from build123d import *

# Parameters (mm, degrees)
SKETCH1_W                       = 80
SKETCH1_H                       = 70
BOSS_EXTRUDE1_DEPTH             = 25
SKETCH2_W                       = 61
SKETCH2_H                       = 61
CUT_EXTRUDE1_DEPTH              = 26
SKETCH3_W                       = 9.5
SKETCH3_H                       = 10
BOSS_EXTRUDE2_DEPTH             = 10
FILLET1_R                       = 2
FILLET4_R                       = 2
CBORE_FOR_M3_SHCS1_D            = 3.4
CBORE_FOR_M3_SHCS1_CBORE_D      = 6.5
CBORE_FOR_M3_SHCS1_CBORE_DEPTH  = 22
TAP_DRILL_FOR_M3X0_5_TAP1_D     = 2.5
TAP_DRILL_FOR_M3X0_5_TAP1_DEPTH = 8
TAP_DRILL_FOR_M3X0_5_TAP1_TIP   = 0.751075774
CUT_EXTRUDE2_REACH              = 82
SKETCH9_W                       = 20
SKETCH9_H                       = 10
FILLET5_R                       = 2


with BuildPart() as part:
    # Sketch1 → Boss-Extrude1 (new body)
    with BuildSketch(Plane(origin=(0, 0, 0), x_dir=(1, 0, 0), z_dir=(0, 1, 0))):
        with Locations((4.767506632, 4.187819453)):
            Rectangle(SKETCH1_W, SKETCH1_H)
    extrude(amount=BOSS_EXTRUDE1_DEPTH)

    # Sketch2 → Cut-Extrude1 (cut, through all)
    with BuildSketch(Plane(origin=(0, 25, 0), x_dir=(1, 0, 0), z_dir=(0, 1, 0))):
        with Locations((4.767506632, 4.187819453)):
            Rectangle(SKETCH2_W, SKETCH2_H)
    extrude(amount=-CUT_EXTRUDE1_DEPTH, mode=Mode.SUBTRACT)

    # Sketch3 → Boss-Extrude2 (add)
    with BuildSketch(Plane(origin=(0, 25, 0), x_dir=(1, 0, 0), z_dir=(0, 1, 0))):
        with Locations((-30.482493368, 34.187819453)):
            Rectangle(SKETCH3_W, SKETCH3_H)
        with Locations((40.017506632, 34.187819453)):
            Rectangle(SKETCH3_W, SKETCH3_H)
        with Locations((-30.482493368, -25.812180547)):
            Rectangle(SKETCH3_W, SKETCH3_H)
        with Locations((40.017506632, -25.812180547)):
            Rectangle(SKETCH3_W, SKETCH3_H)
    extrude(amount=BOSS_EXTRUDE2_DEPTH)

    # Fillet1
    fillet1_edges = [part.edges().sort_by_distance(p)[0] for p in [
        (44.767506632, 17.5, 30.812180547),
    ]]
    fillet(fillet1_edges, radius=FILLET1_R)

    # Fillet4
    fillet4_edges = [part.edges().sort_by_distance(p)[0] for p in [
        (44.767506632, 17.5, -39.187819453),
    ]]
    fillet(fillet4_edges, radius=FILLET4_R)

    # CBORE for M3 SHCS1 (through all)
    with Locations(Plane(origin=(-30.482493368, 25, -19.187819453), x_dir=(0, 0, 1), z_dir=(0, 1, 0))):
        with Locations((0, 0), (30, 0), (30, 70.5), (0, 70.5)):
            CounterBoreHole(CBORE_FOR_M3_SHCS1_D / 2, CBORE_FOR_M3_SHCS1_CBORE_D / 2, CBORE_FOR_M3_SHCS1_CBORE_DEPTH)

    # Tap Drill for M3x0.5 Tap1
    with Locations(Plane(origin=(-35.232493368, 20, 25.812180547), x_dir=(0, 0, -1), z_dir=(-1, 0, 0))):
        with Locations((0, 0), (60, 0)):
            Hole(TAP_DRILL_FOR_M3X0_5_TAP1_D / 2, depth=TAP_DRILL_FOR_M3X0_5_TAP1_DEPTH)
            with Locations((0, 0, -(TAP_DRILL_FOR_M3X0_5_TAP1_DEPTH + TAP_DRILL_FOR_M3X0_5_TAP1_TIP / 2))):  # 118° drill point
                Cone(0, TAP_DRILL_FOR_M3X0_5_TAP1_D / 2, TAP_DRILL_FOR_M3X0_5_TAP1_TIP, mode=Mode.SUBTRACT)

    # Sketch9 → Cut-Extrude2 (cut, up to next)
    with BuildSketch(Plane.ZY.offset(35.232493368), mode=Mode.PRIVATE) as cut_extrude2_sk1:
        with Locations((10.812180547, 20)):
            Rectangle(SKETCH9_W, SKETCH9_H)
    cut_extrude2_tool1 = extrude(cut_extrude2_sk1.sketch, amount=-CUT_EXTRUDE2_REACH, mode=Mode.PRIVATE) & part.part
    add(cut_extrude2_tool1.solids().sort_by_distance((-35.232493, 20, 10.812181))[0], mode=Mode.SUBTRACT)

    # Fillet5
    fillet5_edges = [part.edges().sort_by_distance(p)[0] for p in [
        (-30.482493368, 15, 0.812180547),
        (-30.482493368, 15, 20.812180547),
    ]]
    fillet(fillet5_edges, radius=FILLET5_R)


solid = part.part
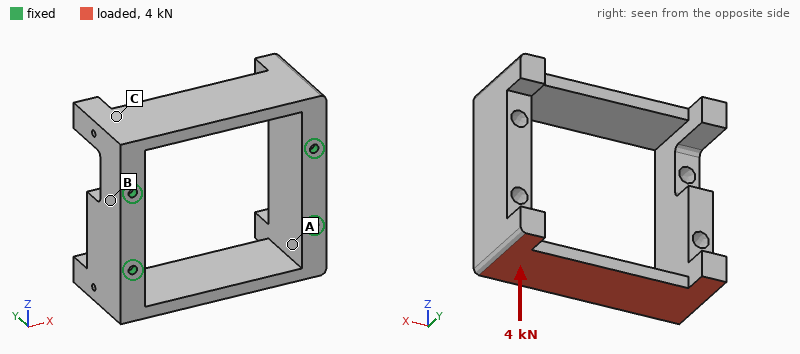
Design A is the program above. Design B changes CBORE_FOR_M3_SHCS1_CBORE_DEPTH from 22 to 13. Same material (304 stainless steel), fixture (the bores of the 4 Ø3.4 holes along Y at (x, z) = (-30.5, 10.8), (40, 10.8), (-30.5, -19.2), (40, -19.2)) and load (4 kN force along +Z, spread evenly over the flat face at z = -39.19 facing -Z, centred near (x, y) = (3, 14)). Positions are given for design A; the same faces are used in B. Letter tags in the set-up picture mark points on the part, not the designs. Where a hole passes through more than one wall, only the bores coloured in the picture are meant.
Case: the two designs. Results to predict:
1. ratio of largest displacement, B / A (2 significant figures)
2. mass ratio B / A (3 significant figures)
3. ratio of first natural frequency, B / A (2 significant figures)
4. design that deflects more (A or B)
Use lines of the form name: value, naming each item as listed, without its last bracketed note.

ratio of largest displacement, B / A: 0.89
mass ratio B / A: 1.02
ratio of first natural frequency, B / A: 1.2
design that deflects more: A
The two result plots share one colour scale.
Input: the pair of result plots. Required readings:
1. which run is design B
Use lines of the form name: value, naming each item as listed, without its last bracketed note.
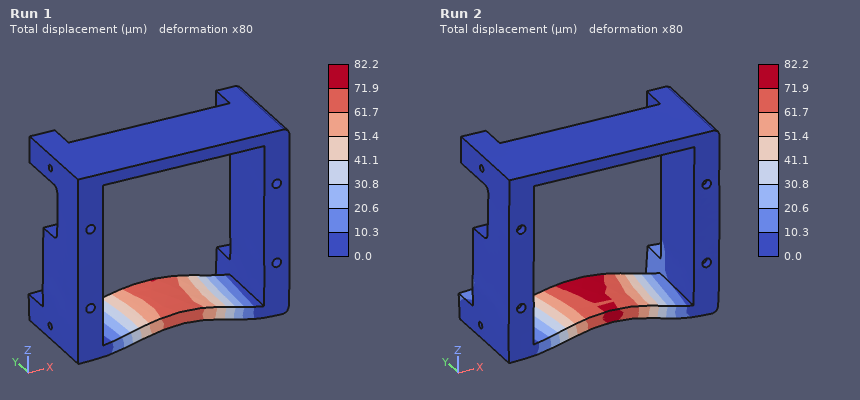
which run is design B: Run 1
